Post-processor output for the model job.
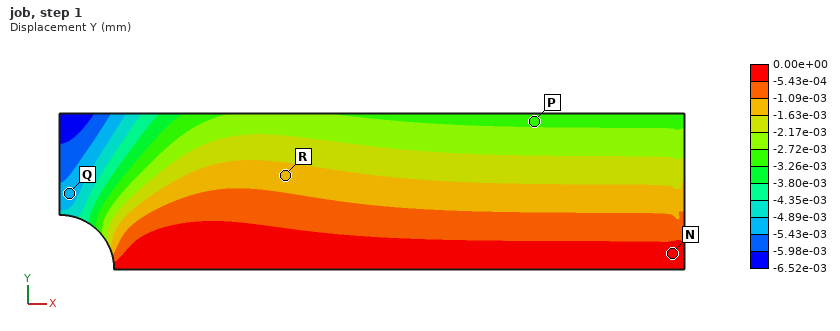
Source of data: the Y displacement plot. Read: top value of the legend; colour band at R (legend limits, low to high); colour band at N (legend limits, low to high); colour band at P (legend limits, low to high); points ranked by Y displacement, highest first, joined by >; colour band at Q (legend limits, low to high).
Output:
0.00e+00 mm
-1.63e-03 to -1.09e-03 mm
-5.43e-04 to 0.00e+00 mm
-3.26e-03 to -2.72e-03 mm
N > R > P > Q
-5.43e-03 to -4.89e-03 mm
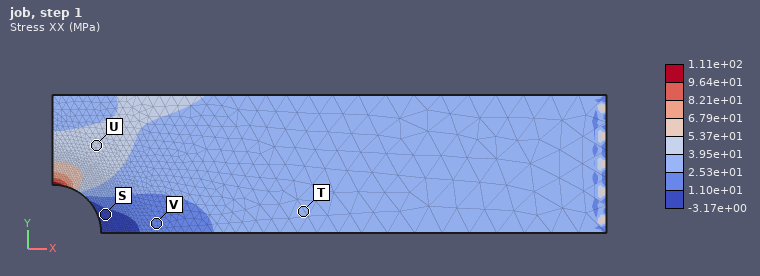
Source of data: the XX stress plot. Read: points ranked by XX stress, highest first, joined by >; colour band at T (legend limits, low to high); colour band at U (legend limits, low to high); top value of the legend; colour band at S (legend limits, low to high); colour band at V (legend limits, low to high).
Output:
U > T > V > S
2.53e+01 to 3.95e+01 MPa
3.95e+01 to 5.37e+01 MPa
1.11e+02 MPa
-3.17e+00 to 1.10e+01 MPa
1.10e+01 to 2.53e+01 MPa
